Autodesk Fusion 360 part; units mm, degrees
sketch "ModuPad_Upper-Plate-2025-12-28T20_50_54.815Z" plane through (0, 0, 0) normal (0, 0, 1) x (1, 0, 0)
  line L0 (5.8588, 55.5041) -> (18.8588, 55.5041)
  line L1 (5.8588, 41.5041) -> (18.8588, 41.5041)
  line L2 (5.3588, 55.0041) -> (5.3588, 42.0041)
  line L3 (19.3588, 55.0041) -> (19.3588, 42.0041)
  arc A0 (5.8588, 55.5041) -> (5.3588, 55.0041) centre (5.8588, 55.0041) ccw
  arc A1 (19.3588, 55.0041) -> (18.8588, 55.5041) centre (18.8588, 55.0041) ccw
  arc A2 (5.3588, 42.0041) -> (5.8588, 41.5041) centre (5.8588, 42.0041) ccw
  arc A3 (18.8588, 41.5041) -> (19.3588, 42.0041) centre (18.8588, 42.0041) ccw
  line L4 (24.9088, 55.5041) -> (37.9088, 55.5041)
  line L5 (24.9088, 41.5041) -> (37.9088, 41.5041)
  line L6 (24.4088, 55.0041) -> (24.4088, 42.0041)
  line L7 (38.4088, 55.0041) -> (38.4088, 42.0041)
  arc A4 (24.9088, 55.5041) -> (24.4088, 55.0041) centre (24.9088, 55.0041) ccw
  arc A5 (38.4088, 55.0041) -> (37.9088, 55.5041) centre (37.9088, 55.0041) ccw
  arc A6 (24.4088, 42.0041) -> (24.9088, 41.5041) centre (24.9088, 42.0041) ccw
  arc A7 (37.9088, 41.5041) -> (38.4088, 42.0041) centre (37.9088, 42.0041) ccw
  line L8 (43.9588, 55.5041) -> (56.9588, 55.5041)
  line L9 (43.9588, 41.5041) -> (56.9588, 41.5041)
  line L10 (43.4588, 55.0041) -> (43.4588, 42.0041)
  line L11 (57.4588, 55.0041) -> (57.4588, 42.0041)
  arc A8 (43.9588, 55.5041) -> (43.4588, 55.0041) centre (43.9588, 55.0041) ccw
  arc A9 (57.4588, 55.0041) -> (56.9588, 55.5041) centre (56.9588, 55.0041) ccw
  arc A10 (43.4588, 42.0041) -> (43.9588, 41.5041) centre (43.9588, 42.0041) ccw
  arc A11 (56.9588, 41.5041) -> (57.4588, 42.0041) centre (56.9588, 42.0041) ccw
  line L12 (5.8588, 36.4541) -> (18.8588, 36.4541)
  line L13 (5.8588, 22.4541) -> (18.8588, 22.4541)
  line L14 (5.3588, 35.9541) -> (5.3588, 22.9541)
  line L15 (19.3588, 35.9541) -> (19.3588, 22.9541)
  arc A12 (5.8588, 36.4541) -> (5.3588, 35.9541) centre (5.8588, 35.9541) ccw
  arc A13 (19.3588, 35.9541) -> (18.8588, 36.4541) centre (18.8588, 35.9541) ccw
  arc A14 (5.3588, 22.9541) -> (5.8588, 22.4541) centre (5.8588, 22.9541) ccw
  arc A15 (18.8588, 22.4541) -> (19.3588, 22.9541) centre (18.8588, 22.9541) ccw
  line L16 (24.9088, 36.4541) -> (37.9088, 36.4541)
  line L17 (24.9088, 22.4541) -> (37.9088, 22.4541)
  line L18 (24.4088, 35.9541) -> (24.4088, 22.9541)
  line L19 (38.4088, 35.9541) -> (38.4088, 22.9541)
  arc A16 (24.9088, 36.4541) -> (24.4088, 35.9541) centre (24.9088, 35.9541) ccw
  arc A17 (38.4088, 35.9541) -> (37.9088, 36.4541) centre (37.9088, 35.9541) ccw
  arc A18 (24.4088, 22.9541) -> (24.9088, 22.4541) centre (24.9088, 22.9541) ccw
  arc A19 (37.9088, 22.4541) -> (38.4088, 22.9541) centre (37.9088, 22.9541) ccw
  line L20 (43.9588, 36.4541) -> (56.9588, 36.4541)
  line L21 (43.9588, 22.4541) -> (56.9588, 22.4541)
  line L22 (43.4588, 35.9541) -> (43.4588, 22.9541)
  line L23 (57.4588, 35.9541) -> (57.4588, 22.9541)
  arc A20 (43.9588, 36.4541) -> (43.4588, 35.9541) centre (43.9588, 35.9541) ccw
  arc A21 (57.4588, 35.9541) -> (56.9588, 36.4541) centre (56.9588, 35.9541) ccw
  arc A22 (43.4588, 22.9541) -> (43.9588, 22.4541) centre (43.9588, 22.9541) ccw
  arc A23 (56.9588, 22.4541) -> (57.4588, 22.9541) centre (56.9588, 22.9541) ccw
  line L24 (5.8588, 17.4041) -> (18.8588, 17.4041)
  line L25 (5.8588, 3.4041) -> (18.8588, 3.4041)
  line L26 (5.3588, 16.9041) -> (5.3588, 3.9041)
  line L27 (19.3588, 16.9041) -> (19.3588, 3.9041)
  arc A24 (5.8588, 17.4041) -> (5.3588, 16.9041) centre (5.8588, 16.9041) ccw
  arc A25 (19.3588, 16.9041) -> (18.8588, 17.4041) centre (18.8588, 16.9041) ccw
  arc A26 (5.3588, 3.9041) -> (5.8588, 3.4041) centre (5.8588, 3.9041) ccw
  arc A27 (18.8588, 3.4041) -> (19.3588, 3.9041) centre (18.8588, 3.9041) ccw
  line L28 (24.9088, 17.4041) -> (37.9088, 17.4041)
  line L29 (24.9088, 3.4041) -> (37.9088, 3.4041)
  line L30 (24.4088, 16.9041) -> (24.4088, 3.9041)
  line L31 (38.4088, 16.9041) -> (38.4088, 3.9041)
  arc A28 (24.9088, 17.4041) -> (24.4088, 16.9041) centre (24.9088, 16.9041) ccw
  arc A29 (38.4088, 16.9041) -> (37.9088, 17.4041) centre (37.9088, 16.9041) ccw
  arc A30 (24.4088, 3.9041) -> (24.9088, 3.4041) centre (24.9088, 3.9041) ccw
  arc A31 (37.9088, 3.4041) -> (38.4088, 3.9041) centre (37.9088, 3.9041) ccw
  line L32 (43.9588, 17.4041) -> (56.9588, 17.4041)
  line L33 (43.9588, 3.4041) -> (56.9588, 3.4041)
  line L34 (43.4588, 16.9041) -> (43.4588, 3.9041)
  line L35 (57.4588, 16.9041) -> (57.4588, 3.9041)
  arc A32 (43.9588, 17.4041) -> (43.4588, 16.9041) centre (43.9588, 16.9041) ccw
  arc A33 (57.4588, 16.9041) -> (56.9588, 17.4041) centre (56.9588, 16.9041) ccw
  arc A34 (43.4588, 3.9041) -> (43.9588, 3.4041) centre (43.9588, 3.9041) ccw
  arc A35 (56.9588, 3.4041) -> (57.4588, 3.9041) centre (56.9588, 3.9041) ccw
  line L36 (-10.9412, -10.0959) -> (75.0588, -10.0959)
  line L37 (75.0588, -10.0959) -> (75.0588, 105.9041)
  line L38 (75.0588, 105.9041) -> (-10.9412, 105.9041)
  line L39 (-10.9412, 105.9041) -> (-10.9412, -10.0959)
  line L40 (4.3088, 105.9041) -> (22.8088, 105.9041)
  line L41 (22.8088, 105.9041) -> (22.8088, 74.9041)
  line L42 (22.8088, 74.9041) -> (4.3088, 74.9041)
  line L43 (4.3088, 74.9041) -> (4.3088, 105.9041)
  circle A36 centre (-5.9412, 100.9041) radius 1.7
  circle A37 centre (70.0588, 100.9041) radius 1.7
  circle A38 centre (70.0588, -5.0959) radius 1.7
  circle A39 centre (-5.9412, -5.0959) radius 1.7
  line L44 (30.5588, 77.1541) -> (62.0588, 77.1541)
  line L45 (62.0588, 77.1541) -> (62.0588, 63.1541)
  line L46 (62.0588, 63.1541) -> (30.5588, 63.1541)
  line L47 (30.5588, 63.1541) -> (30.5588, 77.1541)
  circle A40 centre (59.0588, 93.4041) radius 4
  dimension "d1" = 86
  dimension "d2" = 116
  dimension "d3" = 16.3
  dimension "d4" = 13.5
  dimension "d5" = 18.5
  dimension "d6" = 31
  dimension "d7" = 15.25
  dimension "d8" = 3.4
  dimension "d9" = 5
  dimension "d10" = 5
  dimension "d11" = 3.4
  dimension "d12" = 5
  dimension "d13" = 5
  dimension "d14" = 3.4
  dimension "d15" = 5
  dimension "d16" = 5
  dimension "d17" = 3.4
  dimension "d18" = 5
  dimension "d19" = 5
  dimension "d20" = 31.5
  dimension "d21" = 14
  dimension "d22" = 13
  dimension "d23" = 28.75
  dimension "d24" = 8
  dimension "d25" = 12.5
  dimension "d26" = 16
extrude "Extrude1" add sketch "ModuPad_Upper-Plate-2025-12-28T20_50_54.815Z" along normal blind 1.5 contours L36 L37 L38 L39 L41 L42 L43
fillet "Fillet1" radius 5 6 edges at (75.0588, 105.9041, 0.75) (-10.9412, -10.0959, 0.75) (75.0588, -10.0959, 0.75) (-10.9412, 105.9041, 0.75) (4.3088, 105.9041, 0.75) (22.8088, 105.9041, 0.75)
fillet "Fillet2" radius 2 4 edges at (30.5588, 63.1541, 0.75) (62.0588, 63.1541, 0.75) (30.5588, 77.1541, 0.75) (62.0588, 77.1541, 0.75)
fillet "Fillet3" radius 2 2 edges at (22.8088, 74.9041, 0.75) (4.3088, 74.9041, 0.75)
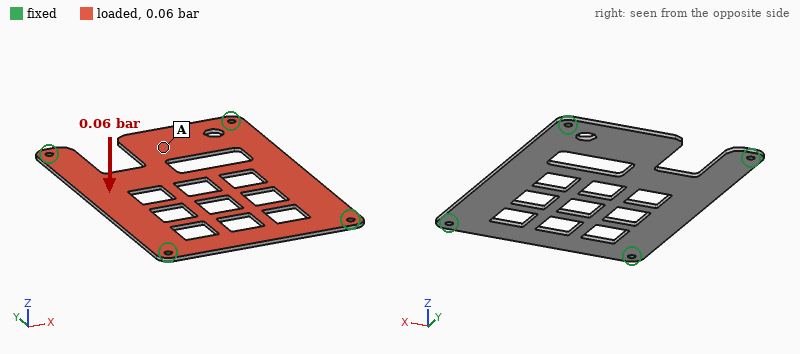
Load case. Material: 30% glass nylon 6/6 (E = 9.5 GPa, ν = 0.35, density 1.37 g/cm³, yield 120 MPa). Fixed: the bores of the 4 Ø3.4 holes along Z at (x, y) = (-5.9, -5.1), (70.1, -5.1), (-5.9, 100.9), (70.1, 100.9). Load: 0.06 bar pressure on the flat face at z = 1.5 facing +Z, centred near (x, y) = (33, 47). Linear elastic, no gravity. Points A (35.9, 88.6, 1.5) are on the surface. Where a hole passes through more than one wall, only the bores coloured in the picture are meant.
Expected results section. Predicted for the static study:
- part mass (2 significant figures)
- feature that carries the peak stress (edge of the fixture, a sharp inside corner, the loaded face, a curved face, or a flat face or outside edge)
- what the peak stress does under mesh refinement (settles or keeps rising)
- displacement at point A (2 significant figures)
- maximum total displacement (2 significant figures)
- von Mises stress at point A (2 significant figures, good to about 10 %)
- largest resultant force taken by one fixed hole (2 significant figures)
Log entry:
15 g
edge of the fixture
keeps rising
0.76 mm
1.4 mm
4.3 MPa
12 N
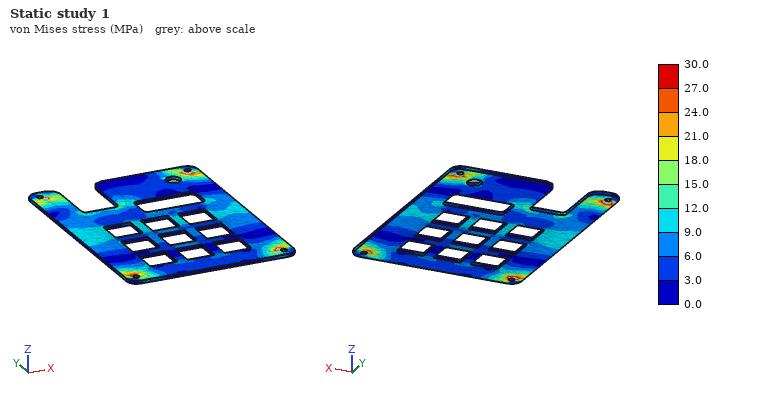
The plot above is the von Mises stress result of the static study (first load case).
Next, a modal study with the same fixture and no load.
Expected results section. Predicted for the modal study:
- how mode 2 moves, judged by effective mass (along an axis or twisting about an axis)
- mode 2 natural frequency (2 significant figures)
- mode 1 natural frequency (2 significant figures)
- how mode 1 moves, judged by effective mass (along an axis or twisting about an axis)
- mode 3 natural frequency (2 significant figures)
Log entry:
twisting about Y
420 Hz
280 Hz
along Z
490 Hz
